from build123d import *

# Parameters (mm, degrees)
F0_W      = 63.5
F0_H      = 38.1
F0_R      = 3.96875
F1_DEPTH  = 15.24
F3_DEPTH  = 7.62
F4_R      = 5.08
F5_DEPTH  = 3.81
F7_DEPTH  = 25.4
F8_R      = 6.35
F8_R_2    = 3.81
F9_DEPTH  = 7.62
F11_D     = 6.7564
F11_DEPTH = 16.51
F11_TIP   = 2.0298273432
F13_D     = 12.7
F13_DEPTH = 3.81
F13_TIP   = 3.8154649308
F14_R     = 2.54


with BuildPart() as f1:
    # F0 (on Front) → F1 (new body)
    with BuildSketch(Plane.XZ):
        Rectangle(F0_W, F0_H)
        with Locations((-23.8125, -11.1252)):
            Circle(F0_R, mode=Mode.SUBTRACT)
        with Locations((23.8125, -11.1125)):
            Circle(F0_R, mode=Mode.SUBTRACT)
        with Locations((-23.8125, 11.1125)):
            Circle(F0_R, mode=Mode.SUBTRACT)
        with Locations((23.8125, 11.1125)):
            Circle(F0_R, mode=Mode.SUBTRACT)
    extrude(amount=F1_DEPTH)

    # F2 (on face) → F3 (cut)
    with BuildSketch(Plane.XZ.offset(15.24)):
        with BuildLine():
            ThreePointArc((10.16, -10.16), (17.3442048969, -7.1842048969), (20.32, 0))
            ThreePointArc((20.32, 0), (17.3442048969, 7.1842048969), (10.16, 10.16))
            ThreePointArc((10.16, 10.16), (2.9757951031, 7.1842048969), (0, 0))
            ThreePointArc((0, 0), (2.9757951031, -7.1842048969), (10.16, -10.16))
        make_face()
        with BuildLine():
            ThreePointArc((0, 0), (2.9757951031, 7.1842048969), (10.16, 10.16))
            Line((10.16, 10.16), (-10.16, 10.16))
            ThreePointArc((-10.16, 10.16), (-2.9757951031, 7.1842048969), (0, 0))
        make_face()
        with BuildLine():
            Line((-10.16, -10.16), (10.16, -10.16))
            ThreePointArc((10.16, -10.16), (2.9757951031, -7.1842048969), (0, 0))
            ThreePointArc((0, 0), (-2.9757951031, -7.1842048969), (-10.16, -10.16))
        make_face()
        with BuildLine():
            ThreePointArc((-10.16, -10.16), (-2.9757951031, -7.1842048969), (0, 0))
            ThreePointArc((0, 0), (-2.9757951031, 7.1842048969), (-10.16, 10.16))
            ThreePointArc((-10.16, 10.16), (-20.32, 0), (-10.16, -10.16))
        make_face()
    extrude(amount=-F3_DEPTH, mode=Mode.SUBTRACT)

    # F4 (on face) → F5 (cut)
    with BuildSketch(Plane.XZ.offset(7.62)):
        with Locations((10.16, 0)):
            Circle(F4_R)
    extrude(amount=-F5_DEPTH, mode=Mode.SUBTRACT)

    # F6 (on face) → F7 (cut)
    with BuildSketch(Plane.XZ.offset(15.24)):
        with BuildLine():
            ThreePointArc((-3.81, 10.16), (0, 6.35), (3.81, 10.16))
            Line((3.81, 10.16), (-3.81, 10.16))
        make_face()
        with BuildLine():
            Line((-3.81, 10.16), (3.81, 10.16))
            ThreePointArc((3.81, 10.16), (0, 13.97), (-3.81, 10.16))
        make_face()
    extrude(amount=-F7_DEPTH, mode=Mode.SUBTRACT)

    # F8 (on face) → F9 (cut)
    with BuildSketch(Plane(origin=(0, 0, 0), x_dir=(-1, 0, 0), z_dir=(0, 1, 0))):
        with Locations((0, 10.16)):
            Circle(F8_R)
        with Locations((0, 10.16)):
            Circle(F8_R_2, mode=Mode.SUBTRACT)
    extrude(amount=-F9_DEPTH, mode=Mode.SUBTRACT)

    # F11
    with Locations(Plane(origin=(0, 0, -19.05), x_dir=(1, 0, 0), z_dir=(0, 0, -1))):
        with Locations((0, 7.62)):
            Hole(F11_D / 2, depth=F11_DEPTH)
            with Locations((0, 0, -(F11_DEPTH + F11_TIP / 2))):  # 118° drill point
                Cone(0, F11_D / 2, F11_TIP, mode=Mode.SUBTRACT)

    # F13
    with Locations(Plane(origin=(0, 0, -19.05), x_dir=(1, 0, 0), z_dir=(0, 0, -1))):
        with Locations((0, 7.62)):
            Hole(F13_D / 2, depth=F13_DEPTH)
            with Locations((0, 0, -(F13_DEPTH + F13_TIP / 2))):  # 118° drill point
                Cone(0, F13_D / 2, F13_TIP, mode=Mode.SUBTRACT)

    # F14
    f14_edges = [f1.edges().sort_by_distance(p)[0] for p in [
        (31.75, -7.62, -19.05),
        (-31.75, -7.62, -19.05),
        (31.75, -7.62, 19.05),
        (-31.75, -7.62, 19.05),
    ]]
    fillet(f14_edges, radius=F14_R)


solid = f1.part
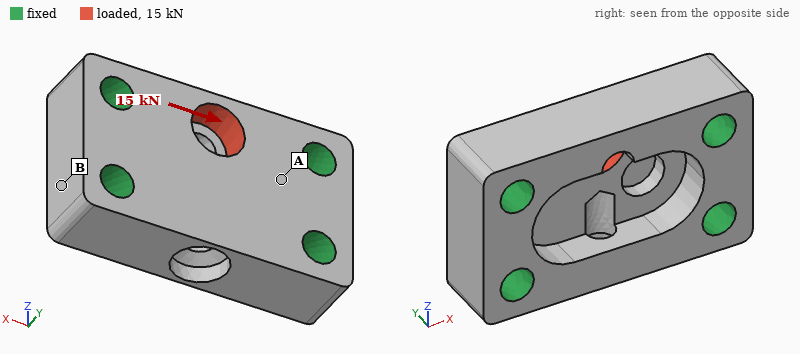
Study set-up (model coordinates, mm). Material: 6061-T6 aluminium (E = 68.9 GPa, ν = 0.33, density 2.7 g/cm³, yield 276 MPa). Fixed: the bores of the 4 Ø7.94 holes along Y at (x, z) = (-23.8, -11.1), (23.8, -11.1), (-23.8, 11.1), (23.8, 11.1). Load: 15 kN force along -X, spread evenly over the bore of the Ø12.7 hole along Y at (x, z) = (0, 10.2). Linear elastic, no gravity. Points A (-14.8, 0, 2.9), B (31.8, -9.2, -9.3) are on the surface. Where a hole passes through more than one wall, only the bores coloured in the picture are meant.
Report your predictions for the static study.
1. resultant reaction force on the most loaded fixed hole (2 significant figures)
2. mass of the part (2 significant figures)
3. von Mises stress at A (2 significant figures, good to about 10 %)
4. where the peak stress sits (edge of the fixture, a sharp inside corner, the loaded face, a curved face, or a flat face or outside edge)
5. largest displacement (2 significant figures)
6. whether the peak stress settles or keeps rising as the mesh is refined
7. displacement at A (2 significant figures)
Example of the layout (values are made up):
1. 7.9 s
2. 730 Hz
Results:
1. 6.1 kN
2. 70 g
3. 25 MPa
4. a sharp inside corner
5. 14 µm
6. keeps rising
7. 4.0 µm
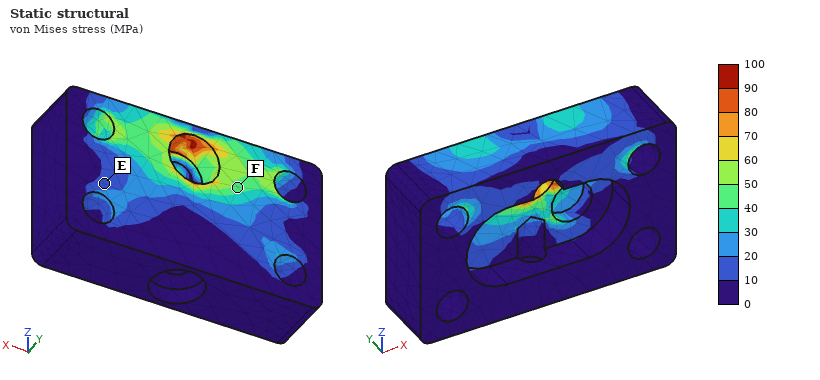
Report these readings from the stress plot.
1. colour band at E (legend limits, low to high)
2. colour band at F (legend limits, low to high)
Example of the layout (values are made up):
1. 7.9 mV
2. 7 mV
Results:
1. 10 to 20 MPa
2. 40 to 50 MPa
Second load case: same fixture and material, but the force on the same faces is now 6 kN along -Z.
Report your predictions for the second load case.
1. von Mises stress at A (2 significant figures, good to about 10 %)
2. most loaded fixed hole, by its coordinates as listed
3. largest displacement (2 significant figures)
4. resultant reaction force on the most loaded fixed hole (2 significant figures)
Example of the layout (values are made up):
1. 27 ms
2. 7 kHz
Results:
1. 21 MPa
2. (-23.8, -11.1)
3. 24 µm
4. 2.0 kN
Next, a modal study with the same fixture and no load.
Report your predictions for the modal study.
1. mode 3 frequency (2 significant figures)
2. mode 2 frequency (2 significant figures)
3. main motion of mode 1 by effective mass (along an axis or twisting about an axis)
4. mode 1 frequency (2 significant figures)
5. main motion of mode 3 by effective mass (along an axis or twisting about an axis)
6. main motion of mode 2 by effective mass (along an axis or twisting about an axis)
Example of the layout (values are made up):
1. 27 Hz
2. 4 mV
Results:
1. 32 kHz
2. 30 kHz
3. along Y
4. 27 kHz
5. along Z
6. along Z
